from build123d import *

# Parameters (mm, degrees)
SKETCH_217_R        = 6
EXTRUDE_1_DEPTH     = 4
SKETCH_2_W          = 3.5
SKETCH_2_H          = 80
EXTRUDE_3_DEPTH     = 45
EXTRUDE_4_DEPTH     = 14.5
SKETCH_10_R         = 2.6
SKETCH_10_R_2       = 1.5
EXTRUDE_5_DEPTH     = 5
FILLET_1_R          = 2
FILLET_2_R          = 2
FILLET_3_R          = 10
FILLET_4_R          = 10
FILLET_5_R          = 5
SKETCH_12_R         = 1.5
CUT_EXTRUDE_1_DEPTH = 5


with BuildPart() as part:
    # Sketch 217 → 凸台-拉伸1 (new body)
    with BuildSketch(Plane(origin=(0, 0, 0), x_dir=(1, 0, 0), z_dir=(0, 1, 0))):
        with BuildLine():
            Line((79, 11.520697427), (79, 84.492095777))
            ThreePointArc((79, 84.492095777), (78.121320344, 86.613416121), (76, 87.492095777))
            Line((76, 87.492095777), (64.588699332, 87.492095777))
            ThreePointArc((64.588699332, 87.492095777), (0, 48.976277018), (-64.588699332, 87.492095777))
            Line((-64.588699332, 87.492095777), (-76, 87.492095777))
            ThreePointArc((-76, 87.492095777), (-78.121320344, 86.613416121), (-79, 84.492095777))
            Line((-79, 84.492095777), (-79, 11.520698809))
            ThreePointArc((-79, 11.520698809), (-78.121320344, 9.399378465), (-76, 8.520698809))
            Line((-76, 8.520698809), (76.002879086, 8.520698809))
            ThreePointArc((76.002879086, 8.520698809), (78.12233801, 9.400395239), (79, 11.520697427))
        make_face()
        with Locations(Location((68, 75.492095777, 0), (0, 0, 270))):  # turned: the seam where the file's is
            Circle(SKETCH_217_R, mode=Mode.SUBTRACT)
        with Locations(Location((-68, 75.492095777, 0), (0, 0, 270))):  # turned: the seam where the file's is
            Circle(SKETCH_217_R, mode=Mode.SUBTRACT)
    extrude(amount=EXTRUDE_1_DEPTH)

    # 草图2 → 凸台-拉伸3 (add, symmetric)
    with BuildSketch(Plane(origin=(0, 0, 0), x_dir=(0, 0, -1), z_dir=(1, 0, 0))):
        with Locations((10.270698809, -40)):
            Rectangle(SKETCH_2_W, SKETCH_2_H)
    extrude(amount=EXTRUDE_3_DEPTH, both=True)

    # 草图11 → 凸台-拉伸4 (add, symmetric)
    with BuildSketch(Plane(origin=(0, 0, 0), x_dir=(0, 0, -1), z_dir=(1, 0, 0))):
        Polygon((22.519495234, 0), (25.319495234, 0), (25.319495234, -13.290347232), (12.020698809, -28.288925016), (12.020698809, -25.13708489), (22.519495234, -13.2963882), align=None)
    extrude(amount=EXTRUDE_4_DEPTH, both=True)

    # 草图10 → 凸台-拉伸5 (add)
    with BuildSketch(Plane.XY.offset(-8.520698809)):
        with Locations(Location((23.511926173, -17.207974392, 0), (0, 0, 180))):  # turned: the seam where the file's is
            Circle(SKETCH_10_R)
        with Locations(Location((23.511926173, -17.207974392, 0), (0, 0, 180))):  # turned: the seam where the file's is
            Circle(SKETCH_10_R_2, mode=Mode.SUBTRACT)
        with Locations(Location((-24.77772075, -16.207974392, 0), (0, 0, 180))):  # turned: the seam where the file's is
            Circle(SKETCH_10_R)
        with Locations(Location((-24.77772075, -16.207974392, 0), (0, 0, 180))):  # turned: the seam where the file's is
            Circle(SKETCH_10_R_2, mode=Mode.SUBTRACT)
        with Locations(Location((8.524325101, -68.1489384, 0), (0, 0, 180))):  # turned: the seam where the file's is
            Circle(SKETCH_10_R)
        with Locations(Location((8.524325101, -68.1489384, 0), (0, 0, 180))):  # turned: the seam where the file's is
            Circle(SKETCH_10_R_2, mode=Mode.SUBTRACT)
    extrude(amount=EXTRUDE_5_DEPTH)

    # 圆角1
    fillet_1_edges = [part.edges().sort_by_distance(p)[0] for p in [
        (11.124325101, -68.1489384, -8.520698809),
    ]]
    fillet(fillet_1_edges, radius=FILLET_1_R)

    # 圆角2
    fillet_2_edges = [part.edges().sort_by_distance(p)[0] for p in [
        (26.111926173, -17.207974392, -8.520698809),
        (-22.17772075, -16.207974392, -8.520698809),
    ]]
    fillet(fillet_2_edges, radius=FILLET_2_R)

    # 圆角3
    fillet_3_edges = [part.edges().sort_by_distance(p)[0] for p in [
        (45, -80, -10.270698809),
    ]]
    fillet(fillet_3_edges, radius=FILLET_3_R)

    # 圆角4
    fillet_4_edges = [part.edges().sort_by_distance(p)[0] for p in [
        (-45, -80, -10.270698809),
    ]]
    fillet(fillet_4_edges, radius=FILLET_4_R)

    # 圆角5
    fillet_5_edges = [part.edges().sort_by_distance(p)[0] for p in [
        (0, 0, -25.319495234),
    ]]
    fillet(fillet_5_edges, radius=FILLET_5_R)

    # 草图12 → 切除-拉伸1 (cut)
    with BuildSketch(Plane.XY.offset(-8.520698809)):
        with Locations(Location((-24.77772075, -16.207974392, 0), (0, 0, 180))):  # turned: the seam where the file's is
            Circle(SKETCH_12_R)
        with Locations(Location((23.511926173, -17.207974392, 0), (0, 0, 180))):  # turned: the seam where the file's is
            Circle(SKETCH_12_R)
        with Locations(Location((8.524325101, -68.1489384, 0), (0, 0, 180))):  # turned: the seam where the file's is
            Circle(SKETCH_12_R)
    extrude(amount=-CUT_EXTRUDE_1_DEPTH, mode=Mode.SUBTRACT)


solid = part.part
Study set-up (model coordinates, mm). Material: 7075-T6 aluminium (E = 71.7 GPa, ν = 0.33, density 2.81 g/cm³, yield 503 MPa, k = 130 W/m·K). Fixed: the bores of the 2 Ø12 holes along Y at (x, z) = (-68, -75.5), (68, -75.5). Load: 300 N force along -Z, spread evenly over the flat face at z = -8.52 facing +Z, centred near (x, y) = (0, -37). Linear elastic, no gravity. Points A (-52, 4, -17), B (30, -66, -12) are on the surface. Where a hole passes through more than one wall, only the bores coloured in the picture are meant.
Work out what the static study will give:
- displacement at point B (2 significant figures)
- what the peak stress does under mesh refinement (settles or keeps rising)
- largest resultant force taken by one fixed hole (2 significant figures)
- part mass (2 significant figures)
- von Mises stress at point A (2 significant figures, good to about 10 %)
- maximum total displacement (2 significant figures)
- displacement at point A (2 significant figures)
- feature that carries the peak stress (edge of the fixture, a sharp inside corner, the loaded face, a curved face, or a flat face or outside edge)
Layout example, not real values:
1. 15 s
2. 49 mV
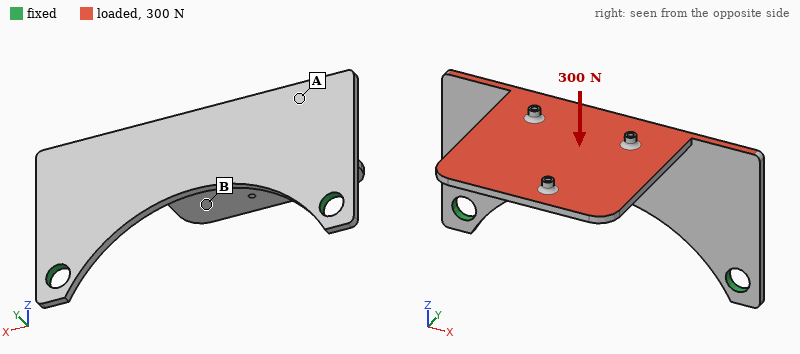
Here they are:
1. 1.6 mm
2. keeps rising
3. 200 N
4. 180 g
5. 26 MPa
6. 2.0 mm
7. 0.57 mm
8. edge of the fixture
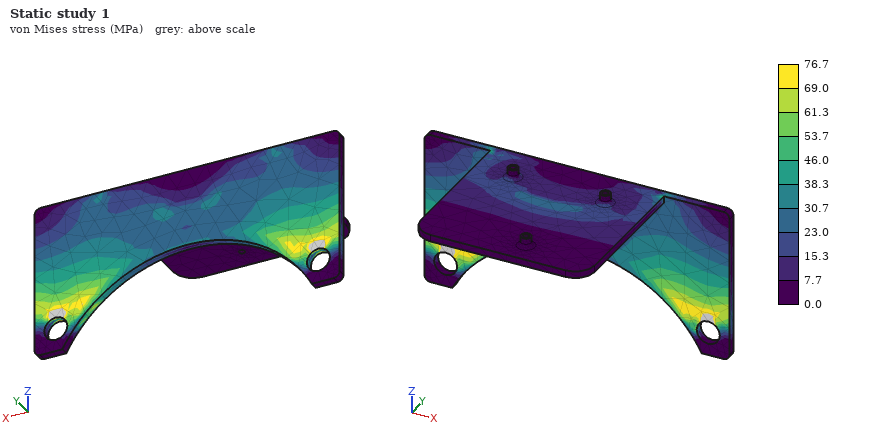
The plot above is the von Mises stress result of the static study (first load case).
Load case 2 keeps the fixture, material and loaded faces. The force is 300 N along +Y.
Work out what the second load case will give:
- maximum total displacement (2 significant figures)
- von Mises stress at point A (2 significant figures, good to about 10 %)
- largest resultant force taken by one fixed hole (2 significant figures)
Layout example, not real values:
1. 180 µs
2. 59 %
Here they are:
1. 1.8 mm
2. 24 MPa
3. 150 N
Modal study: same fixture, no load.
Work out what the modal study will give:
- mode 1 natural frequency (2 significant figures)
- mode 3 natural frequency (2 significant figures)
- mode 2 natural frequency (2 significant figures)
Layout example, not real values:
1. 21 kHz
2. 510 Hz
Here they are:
1. 210 Hz
2. 560 Hz
3. 530 Hz
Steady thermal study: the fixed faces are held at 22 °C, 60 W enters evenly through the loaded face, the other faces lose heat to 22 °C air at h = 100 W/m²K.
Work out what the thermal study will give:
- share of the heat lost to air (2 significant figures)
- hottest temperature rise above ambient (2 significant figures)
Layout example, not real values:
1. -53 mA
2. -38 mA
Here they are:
1. 86 %
2. 41 K
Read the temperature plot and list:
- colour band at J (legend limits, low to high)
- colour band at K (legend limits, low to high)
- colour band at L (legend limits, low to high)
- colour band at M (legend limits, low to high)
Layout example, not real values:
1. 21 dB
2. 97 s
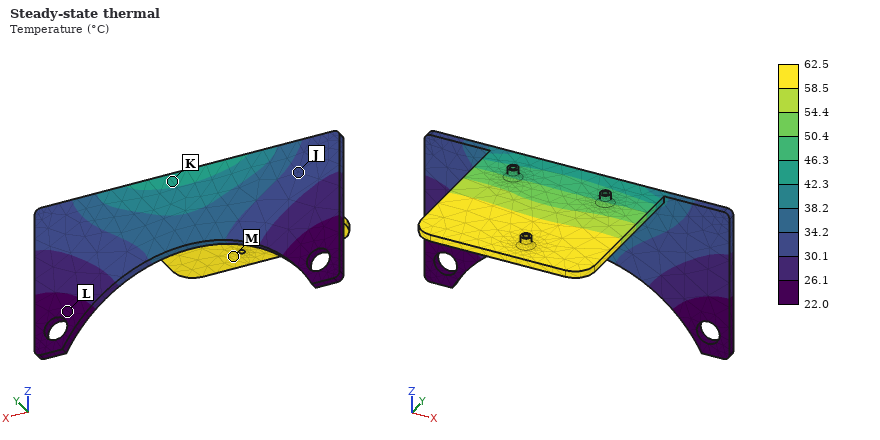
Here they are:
1. 30.1 to 34.2 °C
2. 42.3 to 46.3 °C
3. 22.0 to 26.1 °C
4. 58.5 to 62.5 °C
